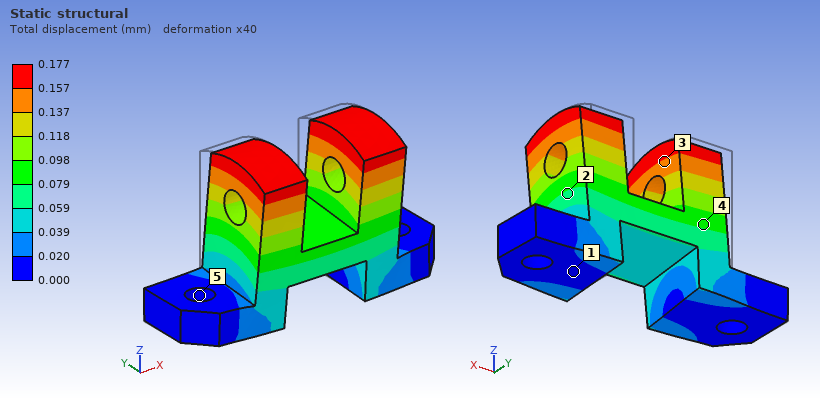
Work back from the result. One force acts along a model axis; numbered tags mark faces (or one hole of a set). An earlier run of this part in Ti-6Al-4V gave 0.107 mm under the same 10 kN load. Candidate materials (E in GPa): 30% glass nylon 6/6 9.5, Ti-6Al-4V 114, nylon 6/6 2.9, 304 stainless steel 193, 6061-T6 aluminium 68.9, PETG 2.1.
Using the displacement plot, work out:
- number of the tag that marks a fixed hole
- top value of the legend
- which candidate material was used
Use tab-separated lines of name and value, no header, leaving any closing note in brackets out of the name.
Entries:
number of the tag that marks a fixed hole	5
top value of the legend	0.177 mm
which candidate material was used	6061-T6 aluminium
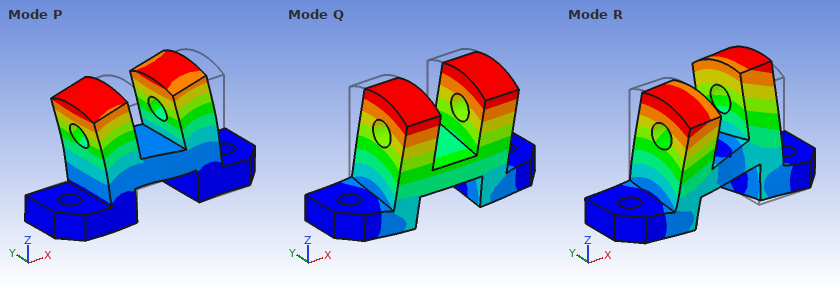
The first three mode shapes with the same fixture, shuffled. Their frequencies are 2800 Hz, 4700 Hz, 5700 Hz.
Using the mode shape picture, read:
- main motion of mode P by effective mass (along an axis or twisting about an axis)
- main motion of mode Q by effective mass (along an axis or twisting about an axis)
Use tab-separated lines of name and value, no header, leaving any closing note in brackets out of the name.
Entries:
main motion of mode P by effective mass	along X
main motion of mode Q by effective mass	along Y
